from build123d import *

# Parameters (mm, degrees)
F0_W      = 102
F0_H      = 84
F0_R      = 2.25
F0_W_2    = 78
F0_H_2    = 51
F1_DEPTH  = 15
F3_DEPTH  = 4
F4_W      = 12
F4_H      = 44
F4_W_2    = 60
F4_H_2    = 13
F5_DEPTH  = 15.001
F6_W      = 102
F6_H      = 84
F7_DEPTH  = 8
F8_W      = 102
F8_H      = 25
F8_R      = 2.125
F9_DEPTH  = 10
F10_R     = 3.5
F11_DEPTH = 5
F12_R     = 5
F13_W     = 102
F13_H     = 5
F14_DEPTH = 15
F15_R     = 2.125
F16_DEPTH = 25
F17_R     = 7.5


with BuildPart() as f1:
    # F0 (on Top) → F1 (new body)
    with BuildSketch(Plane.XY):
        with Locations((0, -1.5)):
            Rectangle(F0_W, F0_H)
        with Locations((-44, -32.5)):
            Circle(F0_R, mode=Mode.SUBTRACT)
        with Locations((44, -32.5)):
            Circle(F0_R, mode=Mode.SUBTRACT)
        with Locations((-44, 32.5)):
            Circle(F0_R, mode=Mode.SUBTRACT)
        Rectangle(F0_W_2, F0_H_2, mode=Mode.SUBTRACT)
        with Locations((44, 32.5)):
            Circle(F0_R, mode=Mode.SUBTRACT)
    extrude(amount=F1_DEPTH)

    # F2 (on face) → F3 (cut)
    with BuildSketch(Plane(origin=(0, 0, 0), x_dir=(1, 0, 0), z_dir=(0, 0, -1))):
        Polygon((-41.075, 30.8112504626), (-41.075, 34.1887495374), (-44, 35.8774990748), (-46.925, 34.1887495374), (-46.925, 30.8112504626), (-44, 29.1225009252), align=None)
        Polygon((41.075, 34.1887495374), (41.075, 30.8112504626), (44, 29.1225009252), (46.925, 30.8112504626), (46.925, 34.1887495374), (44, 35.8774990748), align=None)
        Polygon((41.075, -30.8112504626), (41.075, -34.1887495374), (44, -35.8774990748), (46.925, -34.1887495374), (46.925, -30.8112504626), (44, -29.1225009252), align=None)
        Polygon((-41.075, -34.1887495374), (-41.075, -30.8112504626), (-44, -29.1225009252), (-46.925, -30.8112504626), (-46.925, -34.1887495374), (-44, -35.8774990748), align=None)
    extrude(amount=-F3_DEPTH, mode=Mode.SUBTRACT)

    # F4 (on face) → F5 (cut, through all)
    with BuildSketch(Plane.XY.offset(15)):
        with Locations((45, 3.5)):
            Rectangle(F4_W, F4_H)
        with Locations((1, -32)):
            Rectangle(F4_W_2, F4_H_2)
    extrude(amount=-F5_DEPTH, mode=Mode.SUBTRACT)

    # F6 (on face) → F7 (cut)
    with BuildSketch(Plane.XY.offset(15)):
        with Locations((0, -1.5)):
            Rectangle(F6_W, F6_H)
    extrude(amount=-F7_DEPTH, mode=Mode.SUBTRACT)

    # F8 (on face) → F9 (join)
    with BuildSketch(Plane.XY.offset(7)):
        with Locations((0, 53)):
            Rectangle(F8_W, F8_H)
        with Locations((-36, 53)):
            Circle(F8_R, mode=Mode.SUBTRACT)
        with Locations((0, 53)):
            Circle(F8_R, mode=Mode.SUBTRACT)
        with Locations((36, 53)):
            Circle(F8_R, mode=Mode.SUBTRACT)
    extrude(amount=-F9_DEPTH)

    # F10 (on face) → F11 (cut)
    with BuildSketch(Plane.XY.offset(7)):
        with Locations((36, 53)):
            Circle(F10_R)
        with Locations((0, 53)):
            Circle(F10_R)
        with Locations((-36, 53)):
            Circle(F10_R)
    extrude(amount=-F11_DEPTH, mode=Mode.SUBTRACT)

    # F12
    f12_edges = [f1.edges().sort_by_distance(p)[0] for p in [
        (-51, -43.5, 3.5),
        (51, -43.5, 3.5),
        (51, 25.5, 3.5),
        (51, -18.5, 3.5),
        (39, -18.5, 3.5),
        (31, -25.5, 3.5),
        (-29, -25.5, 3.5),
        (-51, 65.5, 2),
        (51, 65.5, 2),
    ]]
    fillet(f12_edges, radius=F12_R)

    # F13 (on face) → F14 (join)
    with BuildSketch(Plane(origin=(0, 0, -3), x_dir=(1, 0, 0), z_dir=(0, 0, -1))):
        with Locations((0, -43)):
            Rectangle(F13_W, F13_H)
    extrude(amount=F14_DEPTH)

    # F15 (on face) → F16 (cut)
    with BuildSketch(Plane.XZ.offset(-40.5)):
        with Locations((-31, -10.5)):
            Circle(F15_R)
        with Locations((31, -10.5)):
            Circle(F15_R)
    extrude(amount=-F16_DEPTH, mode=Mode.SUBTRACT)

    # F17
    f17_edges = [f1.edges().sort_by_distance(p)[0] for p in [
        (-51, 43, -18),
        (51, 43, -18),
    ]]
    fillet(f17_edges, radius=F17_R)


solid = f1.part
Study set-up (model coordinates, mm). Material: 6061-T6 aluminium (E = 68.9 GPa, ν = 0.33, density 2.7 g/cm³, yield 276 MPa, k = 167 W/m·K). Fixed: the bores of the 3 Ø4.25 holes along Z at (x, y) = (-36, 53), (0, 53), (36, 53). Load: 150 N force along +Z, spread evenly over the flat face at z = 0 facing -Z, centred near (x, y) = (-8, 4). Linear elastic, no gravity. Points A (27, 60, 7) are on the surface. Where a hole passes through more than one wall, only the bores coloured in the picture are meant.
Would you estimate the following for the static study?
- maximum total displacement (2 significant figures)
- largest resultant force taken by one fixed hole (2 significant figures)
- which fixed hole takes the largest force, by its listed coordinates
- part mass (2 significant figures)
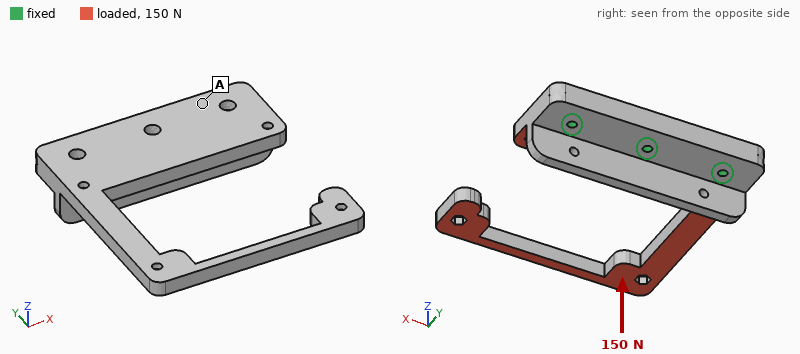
1.5 mm
98 N
(0, 53)
150 g
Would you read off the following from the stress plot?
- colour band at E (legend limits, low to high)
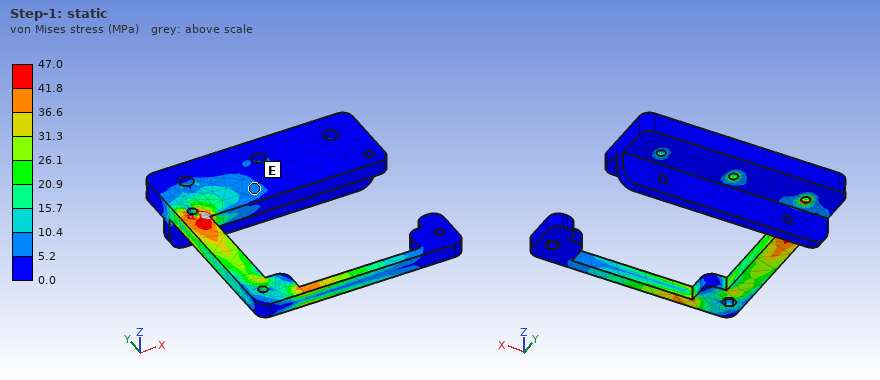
5.2 to 10.4 MPa
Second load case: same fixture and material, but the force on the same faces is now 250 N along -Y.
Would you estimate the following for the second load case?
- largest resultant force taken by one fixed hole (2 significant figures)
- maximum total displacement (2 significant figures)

110 N
1.6 mm
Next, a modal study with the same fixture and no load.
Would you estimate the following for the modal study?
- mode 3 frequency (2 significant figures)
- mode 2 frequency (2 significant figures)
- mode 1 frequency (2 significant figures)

620 Hz
290 Hz
240 Hz
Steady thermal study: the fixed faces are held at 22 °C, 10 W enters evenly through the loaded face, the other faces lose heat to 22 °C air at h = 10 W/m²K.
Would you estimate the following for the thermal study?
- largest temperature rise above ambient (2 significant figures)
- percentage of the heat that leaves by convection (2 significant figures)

35 K
12 %
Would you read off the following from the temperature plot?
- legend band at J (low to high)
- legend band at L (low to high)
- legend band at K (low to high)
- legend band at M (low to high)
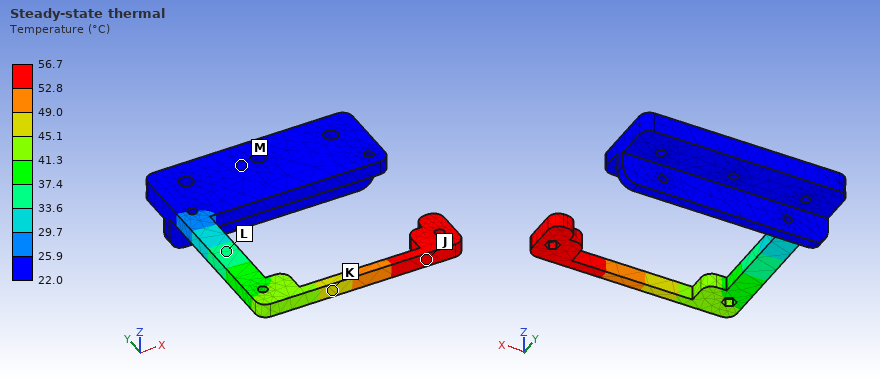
52.8 to 56.7 °C
33.6 to 37.4 °C
45.1 to 49.0 °C
22.0 to 25.9 °C
